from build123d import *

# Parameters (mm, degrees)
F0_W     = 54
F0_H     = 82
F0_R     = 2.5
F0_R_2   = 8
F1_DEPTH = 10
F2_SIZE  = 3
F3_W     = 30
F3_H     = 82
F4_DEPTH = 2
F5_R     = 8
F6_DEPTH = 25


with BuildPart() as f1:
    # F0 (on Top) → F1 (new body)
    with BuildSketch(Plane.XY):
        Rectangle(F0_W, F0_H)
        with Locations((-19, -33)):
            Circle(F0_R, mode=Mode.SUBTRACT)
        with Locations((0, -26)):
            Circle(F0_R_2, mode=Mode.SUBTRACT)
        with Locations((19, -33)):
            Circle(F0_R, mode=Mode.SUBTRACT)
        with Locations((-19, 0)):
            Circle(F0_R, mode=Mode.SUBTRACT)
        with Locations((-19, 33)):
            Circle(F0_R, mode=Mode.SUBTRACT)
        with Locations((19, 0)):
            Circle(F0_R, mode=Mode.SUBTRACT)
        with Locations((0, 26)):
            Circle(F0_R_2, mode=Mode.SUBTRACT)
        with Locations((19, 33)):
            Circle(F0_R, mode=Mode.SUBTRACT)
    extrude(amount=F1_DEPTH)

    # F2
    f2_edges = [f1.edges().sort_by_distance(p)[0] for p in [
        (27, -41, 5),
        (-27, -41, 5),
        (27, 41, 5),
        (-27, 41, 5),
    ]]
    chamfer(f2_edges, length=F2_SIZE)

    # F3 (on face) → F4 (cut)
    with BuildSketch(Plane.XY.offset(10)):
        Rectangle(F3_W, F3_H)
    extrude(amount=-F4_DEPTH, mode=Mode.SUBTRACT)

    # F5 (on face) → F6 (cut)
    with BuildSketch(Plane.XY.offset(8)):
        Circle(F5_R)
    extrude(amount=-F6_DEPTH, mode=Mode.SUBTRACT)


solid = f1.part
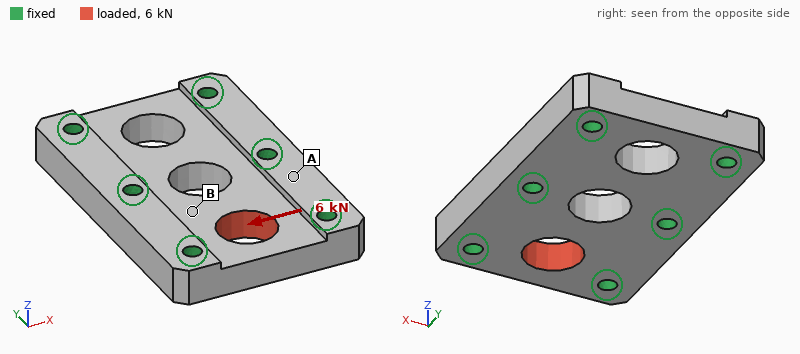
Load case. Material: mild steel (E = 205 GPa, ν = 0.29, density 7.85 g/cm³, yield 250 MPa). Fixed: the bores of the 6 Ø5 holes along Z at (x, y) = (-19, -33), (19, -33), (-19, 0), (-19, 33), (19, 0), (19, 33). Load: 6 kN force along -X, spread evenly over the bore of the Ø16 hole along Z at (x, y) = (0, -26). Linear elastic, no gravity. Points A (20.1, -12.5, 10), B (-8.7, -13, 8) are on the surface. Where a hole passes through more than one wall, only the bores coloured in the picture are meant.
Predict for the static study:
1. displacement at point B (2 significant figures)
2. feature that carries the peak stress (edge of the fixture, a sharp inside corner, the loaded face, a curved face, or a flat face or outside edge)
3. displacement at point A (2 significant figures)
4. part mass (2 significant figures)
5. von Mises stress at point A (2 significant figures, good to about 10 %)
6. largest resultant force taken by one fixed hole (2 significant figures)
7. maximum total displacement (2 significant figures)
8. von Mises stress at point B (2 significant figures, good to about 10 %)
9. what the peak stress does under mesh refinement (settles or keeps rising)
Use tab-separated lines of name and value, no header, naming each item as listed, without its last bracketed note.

displacement at point B	0.90 µm
feature that carries the peak stress	edge of the fixture
displacement at point A	0.72 µm
part mass	260 g
von Mises stress at point A	4.1 MPa
largest resultant force taken by one fixed hole	2.2 kN
maximum total displacement	1.6 µm
von Mises stress at point B	8.6 MPa
what the peak stress does under mesh refinement	keeps rising
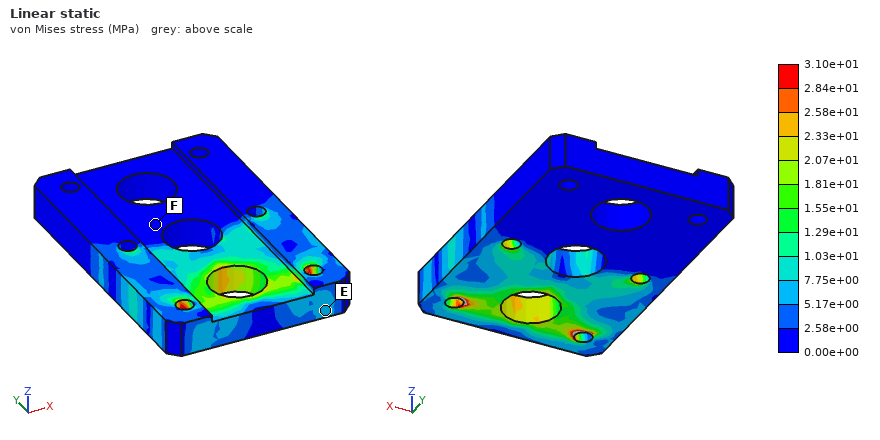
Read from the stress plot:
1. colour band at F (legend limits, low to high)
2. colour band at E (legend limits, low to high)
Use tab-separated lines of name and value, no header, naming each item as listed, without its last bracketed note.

colour band at F	0.00e+00 to 2.58e+00 MPa
colour band at E	5.17e+00 to 7.75e+00 MPa
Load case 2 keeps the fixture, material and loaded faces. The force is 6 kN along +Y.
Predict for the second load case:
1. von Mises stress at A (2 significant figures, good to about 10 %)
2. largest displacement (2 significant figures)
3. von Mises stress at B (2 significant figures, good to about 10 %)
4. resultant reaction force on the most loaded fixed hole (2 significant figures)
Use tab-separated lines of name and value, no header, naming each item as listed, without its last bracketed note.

von Mises stress at A	4.5 MPa
largest displacement	3.9 µm
von Mises stress at B	16 MPa
resultant reaction force on the most loaded fixed hole	1.8 kN
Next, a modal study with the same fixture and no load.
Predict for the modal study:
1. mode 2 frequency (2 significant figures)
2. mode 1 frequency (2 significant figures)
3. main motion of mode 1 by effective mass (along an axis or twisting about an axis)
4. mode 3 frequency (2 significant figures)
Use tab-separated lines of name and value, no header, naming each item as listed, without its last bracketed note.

mode 2 frequency	24 kHz
mode 1 frequency	23 kHz
main motion of mode 1 by effective mass	along Z
mode 3 frequency	30 kHz
